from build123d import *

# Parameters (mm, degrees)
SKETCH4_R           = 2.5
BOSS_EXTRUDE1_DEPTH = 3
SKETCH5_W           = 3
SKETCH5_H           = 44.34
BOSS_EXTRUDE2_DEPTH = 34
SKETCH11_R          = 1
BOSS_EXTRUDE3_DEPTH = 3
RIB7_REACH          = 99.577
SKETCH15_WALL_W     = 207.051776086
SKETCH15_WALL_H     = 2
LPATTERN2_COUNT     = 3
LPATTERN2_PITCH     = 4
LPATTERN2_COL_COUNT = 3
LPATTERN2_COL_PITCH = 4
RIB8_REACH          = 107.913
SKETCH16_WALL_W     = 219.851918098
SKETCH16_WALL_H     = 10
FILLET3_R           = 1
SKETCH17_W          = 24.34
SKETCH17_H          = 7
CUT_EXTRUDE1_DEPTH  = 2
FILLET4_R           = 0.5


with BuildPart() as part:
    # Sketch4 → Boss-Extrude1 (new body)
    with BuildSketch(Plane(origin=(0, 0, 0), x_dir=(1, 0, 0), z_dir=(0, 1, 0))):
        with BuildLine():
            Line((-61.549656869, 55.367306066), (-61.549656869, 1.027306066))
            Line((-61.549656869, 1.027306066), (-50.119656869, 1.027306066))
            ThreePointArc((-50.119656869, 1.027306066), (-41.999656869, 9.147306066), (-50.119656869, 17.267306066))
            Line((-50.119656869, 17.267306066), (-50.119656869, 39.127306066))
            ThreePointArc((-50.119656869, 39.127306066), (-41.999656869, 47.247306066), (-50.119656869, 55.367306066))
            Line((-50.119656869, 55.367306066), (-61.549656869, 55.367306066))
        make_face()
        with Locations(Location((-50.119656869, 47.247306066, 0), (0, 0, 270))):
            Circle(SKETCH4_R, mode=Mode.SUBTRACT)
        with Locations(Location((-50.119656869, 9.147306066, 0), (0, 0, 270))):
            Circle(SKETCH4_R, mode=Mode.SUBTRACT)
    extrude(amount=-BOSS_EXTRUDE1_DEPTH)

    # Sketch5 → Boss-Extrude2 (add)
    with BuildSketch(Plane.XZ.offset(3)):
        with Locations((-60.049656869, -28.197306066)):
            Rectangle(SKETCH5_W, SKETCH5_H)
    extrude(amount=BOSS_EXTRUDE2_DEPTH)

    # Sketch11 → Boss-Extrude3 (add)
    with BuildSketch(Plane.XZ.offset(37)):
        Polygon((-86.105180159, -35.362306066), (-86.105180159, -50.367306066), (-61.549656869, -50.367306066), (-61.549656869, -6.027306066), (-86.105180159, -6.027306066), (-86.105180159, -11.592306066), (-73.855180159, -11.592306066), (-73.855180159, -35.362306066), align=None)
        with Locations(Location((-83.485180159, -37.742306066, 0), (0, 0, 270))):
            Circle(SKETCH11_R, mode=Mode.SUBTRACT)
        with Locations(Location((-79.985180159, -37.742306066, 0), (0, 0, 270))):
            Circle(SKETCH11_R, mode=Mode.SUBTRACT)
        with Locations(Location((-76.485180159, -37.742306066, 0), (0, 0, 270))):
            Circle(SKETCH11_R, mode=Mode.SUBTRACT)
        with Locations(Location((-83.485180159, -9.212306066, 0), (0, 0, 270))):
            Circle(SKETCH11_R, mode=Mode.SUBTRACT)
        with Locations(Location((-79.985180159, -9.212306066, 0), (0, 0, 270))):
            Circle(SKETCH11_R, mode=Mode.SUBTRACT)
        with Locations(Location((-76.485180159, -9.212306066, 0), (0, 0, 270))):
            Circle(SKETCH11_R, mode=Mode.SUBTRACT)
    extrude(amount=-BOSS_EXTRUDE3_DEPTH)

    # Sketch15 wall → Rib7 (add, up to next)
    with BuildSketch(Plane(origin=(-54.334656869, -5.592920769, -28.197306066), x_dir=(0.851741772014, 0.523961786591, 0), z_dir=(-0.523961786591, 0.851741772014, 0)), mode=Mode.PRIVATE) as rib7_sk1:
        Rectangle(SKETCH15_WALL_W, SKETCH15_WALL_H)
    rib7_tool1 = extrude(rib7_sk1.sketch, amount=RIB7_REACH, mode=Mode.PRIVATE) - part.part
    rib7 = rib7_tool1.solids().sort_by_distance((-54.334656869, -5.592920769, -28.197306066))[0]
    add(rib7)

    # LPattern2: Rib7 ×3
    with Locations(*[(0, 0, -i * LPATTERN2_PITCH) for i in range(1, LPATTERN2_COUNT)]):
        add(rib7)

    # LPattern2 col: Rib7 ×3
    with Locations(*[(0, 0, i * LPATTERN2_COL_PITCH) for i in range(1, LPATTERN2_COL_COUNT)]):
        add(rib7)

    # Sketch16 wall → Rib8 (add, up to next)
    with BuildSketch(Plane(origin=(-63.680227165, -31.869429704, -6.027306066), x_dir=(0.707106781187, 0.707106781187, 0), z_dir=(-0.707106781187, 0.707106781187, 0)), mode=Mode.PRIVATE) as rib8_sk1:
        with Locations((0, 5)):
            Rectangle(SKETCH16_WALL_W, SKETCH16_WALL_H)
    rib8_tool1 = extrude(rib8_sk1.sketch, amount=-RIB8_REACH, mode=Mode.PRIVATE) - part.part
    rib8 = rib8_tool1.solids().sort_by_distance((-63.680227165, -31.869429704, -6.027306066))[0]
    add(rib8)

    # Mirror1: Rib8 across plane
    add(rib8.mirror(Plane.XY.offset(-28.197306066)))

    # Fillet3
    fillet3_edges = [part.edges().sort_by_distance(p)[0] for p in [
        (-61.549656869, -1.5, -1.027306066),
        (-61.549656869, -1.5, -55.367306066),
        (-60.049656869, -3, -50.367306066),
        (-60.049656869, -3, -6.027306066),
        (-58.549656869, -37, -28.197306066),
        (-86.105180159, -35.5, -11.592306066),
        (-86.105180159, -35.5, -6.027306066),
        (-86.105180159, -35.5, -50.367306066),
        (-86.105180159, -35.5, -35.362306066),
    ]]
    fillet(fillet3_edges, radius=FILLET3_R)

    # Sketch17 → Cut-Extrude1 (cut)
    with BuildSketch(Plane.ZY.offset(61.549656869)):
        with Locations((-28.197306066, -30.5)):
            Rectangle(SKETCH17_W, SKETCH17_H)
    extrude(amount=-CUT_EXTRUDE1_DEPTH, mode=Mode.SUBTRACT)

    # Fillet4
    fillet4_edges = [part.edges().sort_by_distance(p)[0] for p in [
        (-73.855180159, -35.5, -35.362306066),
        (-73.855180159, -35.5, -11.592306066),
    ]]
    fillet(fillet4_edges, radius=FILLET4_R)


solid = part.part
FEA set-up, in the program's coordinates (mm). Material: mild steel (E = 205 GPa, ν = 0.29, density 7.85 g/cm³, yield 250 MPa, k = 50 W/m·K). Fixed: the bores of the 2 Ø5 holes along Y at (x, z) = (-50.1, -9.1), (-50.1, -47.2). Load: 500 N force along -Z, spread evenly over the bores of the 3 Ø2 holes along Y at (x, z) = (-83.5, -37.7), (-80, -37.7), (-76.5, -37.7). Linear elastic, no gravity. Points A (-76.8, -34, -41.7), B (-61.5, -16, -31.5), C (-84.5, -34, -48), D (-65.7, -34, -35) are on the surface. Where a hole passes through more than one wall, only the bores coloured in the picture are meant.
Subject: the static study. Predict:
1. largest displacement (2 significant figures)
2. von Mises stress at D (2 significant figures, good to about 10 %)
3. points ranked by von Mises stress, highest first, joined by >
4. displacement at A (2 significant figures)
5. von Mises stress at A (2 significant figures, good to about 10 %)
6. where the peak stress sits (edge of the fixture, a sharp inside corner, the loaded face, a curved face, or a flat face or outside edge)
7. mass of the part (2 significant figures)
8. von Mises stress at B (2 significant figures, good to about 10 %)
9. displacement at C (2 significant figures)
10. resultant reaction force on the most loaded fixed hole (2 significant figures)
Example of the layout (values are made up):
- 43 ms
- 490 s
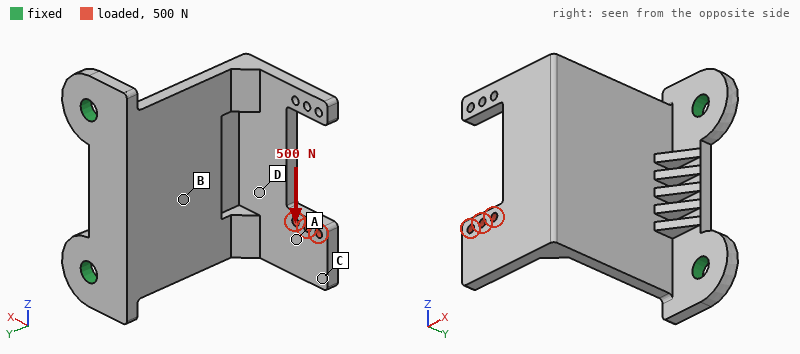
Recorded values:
- 0.23 mm
- 68 MPa
- B > D > A > C
- 0.14 mm
- 38 MPa
- a curved face
- 73 g
- 100 MPa
- 0.21 mm
- 650 N
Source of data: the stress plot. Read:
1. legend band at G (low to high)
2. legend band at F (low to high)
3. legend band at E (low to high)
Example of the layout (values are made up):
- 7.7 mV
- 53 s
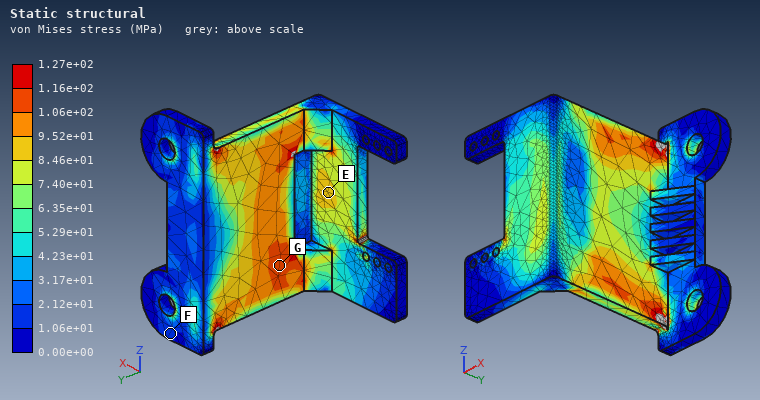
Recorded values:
- 1.06e+02 to 1.16e+02 MPa
- 1.06e+01 to 2.12e+01 MPa
- 8.46e+01 to 9.52e+01 MPa
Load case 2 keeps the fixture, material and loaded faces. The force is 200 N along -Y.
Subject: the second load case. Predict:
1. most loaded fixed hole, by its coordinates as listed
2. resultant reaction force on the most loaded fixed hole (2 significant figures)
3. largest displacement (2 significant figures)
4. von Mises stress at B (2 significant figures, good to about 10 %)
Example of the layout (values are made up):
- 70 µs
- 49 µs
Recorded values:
- (-50.1, -47.2)
- 150 N
- 0.36 mm
- 48 MPa
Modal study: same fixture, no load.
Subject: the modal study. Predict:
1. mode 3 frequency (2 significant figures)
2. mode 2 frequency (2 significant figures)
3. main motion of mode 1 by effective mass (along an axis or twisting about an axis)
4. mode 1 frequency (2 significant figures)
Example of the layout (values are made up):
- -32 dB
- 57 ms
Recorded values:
- 3400 Hz
- 2000 Hz
- along X
- 870 Hz
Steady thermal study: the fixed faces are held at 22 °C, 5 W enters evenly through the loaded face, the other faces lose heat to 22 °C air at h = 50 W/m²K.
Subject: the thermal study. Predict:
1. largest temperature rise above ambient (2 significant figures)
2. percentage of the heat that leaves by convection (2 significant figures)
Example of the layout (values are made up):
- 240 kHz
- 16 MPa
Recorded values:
- 53 K
- 71 %
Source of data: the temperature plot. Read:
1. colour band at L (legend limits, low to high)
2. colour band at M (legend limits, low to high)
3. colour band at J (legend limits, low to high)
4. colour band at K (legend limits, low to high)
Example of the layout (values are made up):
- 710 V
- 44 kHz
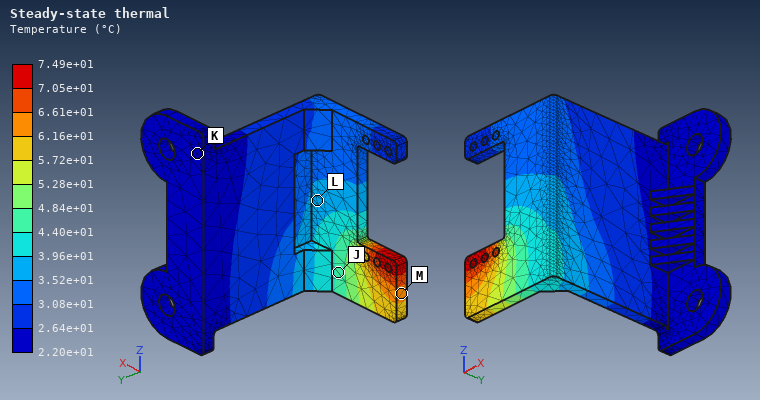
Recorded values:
- 3.52e+01 to 3.96e+01 °C
- 6.16e+01 to 6.61e+01 °C
- 4.40e+01 to 4.84e+01 °C
- 2.20e+01 to 2.64e+01 °C
